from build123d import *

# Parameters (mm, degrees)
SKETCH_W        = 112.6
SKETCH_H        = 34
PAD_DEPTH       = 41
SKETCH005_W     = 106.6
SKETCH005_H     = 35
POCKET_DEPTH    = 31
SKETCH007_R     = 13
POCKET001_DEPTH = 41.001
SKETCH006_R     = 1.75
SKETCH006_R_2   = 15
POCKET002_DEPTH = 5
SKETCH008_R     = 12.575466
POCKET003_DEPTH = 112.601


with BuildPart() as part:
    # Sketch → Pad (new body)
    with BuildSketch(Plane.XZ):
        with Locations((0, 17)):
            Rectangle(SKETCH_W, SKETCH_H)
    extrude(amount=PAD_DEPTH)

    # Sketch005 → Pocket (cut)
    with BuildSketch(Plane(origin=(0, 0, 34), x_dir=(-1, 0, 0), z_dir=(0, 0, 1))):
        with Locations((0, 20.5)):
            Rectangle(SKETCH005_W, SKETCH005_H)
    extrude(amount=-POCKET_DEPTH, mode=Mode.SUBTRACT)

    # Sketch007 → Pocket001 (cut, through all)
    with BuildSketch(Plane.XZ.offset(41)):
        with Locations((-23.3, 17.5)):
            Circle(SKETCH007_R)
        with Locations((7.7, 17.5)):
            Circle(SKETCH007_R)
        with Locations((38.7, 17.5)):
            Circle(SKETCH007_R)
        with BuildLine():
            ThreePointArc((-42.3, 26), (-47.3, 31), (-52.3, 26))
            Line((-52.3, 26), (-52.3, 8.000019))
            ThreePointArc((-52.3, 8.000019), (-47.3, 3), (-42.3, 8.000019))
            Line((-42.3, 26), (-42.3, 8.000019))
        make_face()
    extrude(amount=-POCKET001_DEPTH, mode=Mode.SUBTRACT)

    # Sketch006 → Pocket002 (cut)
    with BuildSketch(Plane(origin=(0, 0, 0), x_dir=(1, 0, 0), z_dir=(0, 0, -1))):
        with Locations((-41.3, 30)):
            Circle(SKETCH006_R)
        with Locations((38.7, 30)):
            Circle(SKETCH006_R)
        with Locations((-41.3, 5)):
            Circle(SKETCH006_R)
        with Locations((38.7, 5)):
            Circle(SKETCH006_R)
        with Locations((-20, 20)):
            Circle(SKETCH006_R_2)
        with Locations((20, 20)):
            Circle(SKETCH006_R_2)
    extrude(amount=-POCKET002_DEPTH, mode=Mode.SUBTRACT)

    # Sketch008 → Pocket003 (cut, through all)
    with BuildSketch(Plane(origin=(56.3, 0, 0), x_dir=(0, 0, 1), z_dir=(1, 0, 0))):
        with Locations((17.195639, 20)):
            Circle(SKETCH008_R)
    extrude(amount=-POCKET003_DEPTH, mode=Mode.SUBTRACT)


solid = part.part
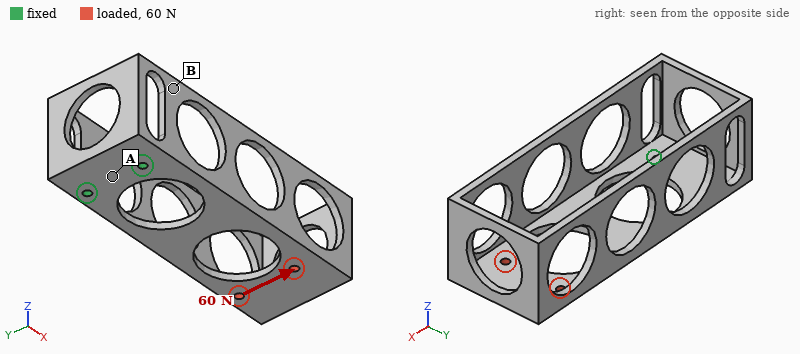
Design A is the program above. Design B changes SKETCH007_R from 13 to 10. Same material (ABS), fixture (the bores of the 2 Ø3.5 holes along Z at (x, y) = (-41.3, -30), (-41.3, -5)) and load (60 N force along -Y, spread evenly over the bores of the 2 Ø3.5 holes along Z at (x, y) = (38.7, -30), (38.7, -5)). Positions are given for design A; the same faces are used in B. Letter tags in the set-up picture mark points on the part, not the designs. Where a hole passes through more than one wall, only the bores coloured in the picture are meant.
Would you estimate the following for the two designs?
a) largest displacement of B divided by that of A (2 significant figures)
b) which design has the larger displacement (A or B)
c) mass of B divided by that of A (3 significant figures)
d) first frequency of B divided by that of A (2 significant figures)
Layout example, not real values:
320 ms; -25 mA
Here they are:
0.90; A; 1.17; 0.98
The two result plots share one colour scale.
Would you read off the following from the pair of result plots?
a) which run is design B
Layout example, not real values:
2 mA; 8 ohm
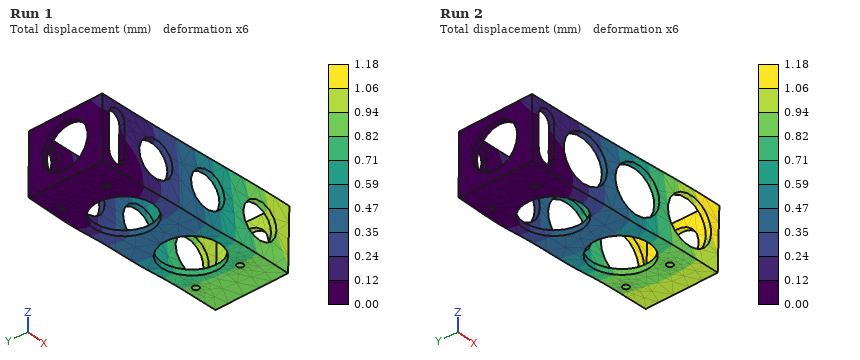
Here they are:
Run 1
